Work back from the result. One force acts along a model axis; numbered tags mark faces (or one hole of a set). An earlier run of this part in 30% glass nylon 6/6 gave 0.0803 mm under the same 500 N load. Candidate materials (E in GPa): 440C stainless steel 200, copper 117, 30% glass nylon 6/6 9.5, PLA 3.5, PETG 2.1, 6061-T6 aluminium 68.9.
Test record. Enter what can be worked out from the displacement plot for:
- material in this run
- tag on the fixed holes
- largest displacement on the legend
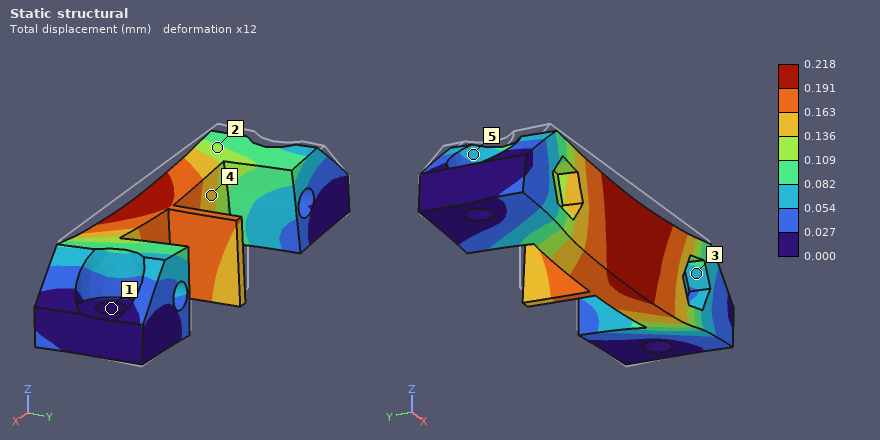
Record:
PLA
1
0.218 mm
